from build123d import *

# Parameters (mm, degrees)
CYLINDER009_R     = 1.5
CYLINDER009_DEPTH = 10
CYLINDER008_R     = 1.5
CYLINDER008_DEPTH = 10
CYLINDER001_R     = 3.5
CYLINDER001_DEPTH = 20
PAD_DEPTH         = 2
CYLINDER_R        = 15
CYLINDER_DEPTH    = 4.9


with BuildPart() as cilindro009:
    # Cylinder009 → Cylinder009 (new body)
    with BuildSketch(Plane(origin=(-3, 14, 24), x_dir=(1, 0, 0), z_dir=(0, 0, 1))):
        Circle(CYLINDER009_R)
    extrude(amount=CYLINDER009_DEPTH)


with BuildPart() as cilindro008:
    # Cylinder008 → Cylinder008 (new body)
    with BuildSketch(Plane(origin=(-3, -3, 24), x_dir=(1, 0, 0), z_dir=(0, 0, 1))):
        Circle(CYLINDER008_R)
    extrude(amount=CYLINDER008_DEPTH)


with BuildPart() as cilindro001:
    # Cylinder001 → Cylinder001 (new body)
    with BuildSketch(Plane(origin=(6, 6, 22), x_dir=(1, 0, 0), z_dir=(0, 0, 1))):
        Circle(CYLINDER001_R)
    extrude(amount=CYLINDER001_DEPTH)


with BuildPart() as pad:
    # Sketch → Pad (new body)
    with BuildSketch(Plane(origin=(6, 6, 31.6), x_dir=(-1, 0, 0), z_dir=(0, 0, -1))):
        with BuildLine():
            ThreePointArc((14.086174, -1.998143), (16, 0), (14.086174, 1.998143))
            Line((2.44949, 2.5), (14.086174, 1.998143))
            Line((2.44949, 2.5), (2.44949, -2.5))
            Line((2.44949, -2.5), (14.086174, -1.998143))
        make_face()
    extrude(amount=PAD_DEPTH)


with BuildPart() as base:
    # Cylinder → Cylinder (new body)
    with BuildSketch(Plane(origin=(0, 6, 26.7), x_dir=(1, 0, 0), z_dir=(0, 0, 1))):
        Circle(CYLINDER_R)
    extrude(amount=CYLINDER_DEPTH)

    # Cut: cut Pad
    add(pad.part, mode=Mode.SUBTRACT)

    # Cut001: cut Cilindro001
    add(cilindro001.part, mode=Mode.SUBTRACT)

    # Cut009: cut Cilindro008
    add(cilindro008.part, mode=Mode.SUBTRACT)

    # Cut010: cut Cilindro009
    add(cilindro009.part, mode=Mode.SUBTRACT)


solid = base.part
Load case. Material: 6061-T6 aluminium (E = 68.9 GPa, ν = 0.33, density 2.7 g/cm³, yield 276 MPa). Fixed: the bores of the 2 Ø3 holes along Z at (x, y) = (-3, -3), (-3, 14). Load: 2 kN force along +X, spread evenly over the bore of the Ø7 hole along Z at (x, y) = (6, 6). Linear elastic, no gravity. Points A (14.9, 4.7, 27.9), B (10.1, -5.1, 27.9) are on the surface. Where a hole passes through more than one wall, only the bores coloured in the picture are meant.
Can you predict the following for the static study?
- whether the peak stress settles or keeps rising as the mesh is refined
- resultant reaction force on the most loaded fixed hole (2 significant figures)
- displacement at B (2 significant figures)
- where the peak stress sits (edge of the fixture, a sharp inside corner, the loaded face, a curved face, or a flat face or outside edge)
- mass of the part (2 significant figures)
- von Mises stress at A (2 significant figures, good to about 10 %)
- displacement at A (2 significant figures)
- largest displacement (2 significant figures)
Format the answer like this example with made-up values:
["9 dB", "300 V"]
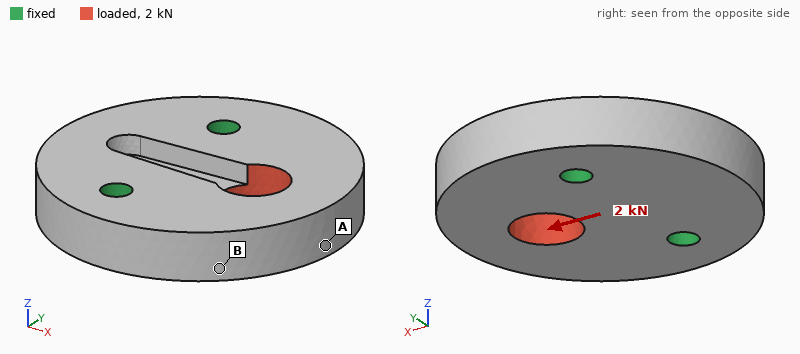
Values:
["keeps rising", "1.1 kN", "1.6 µm", "edge of the fixture", "8.4 g", "25 MPa", "5.8 µm", "7.1 µm"]
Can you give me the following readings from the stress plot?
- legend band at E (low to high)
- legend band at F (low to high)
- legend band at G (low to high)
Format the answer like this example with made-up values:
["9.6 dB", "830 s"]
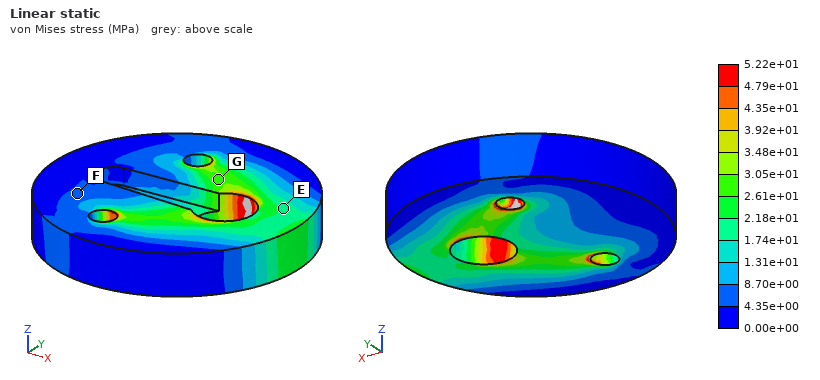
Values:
["1.74e+01 to 2.18e+01 MPa", "4.35e+00 to 8.70e+00 MPa", "2.61e+01 to 3.05e+01 MPa"]
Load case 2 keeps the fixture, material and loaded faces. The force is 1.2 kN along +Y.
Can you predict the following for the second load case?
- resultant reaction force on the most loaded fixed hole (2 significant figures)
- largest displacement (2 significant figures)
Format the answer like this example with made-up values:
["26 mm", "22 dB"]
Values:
["810 N", "9.5 µm"]
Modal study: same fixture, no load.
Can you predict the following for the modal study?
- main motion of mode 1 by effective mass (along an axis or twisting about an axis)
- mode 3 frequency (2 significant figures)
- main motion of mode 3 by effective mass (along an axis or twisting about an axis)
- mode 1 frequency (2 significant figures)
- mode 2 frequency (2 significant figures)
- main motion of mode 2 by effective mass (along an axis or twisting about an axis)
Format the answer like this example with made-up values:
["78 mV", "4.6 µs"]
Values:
["along Z", "28 kHz", "along Z", "14 kHz", "27 kHz", "twisting about X"]
